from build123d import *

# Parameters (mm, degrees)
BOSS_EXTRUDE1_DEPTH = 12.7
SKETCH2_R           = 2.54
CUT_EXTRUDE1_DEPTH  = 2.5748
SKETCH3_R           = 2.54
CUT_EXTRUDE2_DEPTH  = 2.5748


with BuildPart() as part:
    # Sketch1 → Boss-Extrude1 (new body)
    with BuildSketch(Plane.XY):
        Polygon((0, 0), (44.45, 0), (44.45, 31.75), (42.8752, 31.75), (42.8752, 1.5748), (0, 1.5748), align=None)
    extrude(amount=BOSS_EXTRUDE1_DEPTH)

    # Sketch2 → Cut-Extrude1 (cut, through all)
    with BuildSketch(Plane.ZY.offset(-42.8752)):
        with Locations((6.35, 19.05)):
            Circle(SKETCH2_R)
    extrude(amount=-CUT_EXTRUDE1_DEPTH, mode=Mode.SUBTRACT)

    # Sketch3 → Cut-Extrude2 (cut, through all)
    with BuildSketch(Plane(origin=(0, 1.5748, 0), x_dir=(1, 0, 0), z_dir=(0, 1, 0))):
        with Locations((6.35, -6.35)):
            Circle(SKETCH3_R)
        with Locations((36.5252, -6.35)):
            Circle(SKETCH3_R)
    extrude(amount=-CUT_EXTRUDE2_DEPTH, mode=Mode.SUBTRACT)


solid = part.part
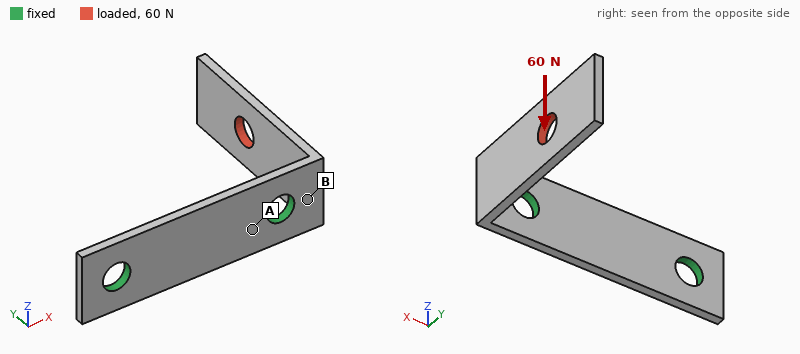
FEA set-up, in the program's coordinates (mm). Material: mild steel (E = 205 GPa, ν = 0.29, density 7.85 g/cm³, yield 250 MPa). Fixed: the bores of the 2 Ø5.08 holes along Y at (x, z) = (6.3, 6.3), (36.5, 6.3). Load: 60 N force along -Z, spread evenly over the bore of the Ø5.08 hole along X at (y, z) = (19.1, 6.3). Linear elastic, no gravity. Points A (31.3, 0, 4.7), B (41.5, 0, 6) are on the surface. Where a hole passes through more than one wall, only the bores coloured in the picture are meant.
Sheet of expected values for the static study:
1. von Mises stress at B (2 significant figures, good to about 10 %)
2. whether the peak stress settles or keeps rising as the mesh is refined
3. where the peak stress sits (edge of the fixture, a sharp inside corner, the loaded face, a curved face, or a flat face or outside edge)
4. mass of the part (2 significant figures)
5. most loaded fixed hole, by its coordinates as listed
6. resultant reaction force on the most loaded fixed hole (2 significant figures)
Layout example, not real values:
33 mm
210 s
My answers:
120 MPa
keeps rising
edge of the fixture
11 g
(36.5, 6.3)
64 N
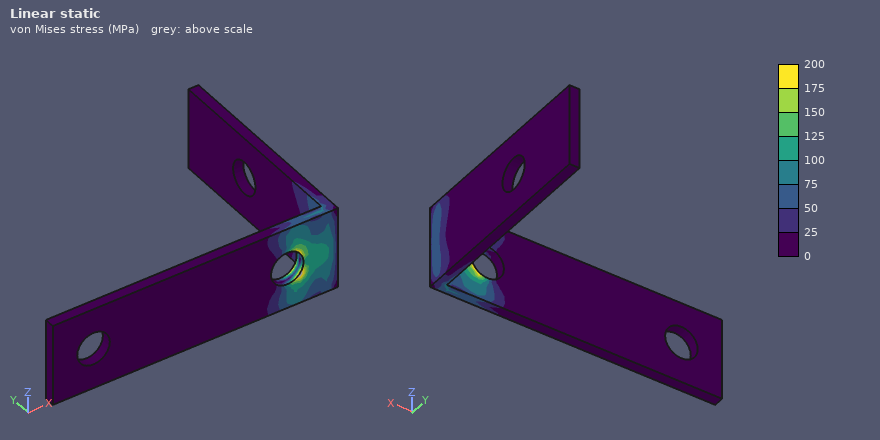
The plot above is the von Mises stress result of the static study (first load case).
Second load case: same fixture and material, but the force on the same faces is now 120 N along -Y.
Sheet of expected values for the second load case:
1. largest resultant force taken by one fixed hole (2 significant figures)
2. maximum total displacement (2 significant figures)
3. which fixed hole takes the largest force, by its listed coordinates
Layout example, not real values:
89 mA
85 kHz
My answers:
120 N
63 µm
(36.5, 6.3)
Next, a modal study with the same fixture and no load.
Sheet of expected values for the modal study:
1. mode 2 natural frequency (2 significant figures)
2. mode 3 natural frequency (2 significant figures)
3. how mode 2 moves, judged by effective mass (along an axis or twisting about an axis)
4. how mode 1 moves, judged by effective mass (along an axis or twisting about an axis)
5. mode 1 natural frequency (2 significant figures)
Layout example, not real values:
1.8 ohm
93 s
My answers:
2400 Hz
6300 Hz
along Z
along X
1100 Hz
